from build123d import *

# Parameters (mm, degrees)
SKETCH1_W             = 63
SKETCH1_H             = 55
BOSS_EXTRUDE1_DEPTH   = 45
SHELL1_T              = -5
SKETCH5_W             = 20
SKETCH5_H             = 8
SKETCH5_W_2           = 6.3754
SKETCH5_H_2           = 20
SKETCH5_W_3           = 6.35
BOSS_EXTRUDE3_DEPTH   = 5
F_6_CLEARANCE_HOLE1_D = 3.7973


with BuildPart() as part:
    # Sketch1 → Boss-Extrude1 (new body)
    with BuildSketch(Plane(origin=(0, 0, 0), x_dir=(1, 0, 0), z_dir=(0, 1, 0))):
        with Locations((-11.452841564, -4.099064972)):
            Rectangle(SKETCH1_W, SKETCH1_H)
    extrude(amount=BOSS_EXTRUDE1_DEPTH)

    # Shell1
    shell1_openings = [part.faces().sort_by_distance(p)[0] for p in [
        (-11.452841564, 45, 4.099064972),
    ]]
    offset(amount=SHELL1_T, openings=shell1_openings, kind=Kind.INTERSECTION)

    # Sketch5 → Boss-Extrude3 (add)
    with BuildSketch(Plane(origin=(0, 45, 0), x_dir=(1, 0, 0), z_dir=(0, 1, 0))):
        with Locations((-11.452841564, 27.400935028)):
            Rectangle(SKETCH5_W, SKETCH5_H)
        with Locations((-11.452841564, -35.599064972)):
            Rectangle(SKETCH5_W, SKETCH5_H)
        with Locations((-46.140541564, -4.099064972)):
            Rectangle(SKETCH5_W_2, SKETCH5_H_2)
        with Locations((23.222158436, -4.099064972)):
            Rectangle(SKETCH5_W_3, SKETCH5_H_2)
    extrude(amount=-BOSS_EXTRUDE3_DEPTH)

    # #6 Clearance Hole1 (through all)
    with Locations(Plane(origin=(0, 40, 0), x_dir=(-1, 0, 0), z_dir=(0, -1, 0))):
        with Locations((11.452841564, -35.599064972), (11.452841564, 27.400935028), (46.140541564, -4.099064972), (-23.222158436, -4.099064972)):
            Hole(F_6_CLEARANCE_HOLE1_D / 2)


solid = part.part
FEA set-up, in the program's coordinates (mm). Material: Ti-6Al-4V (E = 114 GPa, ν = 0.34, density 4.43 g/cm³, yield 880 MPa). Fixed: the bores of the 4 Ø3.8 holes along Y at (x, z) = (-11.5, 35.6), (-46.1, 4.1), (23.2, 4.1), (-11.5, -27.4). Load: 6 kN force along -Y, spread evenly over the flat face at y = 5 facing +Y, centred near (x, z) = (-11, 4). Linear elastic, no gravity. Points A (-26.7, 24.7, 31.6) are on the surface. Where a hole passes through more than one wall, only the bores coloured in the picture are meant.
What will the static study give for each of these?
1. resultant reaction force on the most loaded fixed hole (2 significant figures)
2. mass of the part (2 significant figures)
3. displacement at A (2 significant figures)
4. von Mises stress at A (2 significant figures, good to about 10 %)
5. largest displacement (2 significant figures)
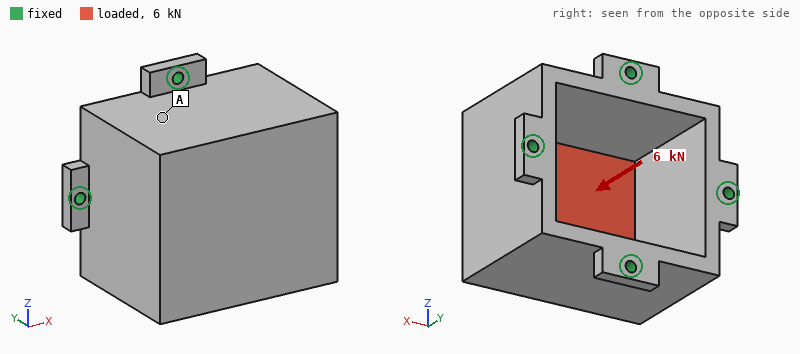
1.6 kN
280 g
7.9 µm
8.6 MPa
39 µm
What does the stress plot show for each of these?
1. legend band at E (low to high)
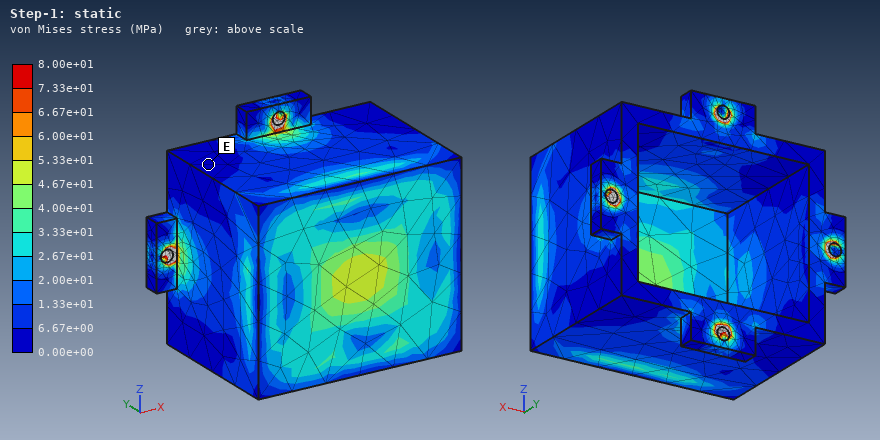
0.00e+00 to 6.67e+00 MPa
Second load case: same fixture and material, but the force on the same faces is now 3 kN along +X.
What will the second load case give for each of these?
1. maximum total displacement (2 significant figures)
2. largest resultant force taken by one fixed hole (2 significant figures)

23 µm
1.8 kN
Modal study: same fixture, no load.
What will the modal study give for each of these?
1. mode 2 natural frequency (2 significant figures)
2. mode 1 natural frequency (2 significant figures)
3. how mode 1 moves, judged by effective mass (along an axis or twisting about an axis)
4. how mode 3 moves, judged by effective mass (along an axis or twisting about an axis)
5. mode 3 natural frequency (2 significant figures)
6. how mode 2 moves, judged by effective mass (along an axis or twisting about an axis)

4800 Hz
4200 Hz
along Z
along Y
8300 Hz
along X
